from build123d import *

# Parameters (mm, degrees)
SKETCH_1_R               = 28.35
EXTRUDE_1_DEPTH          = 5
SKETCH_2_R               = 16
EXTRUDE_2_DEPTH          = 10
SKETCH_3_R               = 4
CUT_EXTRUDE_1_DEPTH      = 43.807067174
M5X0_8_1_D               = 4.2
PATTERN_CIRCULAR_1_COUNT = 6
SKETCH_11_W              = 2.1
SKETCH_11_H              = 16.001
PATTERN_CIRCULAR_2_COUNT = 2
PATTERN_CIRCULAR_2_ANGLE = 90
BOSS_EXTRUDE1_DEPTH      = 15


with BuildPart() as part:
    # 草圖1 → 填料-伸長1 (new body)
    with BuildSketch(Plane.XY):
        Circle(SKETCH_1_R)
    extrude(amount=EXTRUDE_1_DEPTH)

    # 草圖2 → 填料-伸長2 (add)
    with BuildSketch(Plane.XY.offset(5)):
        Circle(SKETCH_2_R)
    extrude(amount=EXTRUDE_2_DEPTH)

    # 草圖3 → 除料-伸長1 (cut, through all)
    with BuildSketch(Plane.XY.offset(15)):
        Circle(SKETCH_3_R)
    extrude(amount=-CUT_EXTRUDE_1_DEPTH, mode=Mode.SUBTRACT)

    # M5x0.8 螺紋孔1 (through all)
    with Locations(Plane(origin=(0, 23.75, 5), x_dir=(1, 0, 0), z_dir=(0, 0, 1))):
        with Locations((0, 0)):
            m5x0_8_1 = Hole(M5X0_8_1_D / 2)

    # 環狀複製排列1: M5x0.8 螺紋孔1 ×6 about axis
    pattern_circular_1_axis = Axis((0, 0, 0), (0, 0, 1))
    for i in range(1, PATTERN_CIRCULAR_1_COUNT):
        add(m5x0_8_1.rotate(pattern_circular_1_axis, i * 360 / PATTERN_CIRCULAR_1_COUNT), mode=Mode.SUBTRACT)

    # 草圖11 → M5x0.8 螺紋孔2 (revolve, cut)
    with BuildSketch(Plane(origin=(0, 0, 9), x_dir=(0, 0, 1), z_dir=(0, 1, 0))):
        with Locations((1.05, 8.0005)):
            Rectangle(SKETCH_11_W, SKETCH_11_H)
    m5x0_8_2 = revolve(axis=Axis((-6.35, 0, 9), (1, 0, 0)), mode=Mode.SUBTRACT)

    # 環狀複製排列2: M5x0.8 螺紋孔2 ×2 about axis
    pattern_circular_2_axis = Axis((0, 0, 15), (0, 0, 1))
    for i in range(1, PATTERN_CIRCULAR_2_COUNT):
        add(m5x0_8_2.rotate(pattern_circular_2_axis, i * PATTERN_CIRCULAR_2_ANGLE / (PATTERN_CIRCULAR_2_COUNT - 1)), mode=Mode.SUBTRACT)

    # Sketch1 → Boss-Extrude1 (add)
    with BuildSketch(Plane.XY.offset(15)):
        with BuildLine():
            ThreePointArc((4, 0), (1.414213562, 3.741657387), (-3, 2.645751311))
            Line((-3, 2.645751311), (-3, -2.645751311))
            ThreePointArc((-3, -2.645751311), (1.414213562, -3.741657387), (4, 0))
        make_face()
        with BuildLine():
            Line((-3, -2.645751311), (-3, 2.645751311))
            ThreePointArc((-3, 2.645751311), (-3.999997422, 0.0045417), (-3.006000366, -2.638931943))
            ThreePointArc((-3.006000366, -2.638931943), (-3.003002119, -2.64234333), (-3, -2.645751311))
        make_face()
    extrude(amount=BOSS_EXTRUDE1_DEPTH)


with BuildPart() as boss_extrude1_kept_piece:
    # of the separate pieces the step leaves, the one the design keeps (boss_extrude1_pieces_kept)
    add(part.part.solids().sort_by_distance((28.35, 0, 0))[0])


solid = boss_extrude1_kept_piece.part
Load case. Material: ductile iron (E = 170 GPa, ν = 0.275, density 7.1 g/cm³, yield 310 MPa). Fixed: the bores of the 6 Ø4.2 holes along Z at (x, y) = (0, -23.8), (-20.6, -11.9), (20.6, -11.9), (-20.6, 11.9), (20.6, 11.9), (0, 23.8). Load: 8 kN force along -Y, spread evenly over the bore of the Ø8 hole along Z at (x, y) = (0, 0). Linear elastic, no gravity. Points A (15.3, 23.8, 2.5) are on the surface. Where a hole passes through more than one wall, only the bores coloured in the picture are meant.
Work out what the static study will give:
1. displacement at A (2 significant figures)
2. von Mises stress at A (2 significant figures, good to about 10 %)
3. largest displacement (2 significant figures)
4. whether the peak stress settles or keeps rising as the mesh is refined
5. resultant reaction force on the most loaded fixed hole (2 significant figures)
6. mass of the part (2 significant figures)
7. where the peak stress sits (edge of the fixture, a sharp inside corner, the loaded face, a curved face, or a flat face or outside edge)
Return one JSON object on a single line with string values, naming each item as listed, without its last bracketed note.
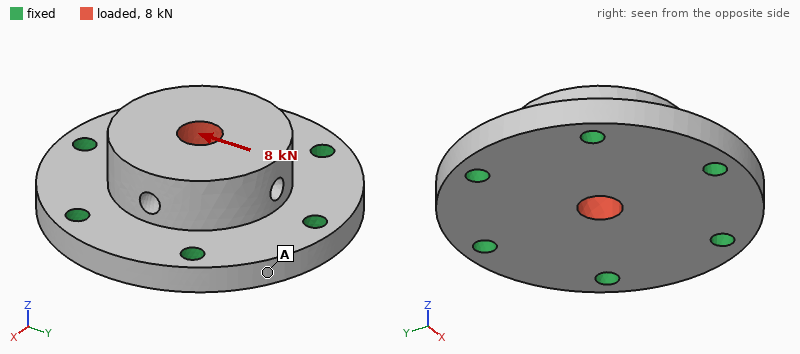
{"displacement at A": "1.2 µm", "von Mises stress at A": "13 MPa", "largest displacement": "5.4 µm", "whether the peak stress settles or keeps rising as the mesh is refined": "keeps rising", "resultant reaction force on the most loaded fixed hole": "2.1 kN", "mass of the part": "140 g", "where the peak stress sits": "edge of the fixture"}
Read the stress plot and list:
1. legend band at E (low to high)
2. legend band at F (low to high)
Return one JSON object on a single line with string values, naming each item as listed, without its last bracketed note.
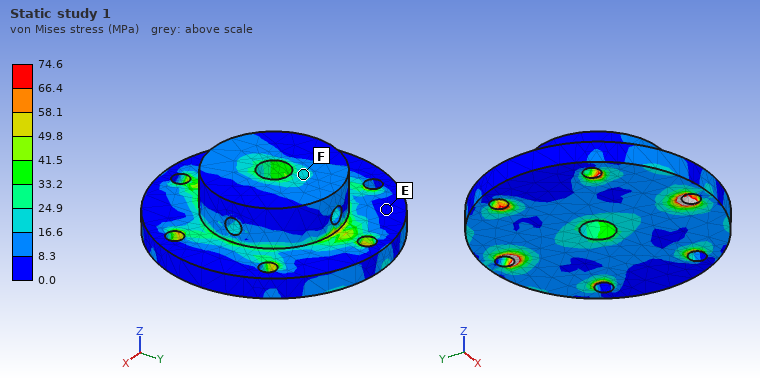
{"legend band at E": "0.0 to 8.3 MPa", "legend band at F": "16.6 to 24.9 MPa"}
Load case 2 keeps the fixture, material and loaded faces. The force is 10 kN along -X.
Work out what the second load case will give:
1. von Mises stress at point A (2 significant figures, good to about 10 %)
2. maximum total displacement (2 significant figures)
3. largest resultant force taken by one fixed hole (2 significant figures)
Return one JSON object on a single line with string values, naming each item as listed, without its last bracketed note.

{"von Mises stress at point A": "9.9 MPa", "maximum total displacement": "6.7 µm", "largest resultant force taken by one fixed hole": "2.3 kN"}
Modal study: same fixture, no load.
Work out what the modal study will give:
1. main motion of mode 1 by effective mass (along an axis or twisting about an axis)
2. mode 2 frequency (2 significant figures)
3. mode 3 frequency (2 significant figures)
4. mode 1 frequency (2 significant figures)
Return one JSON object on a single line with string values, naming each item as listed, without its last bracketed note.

{"main motion of mode 1 by effective mass": "along Z", "mode 2 frequency": "23 kHz", "mode 3 frequency": "23 kHz", "mode 1 frequency": "18 kHz"}
